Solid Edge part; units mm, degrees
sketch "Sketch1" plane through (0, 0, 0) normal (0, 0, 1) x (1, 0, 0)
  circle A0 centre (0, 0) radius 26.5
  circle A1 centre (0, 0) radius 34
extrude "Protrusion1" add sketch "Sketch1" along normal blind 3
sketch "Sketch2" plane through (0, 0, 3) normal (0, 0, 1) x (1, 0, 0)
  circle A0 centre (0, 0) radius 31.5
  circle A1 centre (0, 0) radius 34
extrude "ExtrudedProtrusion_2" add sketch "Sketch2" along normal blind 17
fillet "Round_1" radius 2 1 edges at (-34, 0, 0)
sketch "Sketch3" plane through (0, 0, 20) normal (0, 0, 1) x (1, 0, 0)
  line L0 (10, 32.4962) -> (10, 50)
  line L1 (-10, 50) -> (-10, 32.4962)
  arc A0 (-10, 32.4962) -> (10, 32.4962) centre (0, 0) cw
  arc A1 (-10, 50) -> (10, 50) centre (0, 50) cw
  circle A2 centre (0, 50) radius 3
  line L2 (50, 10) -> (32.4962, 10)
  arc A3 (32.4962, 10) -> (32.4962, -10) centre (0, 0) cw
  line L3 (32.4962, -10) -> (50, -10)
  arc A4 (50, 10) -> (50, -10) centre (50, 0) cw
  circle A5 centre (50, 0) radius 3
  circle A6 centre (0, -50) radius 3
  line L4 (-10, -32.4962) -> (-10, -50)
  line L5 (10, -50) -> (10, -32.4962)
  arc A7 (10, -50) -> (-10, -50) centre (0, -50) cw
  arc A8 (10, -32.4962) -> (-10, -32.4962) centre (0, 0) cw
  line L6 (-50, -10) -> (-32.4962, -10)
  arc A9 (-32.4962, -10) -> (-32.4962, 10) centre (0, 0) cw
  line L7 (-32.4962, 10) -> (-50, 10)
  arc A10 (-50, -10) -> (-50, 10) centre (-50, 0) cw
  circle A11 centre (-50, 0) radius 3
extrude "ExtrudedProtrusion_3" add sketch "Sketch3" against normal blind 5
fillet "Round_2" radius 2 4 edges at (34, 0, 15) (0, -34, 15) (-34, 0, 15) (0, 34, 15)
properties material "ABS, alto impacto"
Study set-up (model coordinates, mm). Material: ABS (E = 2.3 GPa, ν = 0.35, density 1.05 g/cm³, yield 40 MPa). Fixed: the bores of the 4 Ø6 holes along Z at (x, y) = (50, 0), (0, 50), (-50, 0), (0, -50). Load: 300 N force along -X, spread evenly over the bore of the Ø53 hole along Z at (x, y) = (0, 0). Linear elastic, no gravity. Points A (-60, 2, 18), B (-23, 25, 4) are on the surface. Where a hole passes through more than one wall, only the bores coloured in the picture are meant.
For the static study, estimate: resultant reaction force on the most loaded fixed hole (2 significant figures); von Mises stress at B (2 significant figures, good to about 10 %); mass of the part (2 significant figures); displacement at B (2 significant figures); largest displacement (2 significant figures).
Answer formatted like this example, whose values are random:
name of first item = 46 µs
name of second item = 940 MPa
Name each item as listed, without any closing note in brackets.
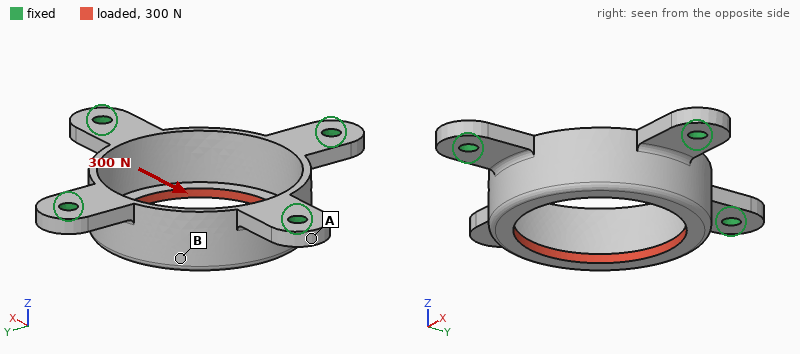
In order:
resultant reaction force on the most loaded fixed hole = 91 N
von Mises stress at B = 2.0 MPa
mass of the part = 23 g
displacement at B = 0.13 mm
largest displacement = 0.15 mm
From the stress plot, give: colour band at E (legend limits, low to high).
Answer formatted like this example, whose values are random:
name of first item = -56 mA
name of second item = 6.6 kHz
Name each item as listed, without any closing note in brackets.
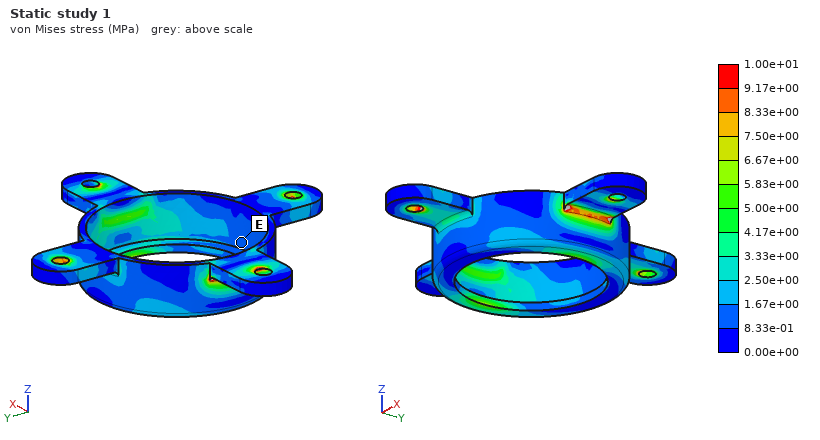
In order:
colour band at E = 8.33e-01 to 1.67e+00 MPa
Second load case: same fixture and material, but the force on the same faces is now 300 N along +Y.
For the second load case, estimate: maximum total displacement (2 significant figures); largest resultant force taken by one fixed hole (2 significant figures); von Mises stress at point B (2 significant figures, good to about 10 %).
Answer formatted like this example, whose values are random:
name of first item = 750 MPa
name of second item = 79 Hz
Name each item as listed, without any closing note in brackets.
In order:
maximum total displacement = 0.15 mm
largest resultant force taken by one fixed hole = 91 N
von Mises stress at point B = 1.9 MPa
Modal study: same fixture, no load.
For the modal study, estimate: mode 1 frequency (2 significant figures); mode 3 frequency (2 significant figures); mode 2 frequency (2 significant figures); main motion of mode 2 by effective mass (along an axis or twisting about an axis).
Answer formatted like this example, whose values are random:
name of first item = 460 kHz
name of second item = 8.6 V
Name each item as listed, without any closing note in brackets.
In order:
mode 1 frequency = 1700 Hz
mode 3 frequency = 2000 Hz
mode 2 frequency = 1900 Hz
main motion of mode 2 by effective mass = along Z
